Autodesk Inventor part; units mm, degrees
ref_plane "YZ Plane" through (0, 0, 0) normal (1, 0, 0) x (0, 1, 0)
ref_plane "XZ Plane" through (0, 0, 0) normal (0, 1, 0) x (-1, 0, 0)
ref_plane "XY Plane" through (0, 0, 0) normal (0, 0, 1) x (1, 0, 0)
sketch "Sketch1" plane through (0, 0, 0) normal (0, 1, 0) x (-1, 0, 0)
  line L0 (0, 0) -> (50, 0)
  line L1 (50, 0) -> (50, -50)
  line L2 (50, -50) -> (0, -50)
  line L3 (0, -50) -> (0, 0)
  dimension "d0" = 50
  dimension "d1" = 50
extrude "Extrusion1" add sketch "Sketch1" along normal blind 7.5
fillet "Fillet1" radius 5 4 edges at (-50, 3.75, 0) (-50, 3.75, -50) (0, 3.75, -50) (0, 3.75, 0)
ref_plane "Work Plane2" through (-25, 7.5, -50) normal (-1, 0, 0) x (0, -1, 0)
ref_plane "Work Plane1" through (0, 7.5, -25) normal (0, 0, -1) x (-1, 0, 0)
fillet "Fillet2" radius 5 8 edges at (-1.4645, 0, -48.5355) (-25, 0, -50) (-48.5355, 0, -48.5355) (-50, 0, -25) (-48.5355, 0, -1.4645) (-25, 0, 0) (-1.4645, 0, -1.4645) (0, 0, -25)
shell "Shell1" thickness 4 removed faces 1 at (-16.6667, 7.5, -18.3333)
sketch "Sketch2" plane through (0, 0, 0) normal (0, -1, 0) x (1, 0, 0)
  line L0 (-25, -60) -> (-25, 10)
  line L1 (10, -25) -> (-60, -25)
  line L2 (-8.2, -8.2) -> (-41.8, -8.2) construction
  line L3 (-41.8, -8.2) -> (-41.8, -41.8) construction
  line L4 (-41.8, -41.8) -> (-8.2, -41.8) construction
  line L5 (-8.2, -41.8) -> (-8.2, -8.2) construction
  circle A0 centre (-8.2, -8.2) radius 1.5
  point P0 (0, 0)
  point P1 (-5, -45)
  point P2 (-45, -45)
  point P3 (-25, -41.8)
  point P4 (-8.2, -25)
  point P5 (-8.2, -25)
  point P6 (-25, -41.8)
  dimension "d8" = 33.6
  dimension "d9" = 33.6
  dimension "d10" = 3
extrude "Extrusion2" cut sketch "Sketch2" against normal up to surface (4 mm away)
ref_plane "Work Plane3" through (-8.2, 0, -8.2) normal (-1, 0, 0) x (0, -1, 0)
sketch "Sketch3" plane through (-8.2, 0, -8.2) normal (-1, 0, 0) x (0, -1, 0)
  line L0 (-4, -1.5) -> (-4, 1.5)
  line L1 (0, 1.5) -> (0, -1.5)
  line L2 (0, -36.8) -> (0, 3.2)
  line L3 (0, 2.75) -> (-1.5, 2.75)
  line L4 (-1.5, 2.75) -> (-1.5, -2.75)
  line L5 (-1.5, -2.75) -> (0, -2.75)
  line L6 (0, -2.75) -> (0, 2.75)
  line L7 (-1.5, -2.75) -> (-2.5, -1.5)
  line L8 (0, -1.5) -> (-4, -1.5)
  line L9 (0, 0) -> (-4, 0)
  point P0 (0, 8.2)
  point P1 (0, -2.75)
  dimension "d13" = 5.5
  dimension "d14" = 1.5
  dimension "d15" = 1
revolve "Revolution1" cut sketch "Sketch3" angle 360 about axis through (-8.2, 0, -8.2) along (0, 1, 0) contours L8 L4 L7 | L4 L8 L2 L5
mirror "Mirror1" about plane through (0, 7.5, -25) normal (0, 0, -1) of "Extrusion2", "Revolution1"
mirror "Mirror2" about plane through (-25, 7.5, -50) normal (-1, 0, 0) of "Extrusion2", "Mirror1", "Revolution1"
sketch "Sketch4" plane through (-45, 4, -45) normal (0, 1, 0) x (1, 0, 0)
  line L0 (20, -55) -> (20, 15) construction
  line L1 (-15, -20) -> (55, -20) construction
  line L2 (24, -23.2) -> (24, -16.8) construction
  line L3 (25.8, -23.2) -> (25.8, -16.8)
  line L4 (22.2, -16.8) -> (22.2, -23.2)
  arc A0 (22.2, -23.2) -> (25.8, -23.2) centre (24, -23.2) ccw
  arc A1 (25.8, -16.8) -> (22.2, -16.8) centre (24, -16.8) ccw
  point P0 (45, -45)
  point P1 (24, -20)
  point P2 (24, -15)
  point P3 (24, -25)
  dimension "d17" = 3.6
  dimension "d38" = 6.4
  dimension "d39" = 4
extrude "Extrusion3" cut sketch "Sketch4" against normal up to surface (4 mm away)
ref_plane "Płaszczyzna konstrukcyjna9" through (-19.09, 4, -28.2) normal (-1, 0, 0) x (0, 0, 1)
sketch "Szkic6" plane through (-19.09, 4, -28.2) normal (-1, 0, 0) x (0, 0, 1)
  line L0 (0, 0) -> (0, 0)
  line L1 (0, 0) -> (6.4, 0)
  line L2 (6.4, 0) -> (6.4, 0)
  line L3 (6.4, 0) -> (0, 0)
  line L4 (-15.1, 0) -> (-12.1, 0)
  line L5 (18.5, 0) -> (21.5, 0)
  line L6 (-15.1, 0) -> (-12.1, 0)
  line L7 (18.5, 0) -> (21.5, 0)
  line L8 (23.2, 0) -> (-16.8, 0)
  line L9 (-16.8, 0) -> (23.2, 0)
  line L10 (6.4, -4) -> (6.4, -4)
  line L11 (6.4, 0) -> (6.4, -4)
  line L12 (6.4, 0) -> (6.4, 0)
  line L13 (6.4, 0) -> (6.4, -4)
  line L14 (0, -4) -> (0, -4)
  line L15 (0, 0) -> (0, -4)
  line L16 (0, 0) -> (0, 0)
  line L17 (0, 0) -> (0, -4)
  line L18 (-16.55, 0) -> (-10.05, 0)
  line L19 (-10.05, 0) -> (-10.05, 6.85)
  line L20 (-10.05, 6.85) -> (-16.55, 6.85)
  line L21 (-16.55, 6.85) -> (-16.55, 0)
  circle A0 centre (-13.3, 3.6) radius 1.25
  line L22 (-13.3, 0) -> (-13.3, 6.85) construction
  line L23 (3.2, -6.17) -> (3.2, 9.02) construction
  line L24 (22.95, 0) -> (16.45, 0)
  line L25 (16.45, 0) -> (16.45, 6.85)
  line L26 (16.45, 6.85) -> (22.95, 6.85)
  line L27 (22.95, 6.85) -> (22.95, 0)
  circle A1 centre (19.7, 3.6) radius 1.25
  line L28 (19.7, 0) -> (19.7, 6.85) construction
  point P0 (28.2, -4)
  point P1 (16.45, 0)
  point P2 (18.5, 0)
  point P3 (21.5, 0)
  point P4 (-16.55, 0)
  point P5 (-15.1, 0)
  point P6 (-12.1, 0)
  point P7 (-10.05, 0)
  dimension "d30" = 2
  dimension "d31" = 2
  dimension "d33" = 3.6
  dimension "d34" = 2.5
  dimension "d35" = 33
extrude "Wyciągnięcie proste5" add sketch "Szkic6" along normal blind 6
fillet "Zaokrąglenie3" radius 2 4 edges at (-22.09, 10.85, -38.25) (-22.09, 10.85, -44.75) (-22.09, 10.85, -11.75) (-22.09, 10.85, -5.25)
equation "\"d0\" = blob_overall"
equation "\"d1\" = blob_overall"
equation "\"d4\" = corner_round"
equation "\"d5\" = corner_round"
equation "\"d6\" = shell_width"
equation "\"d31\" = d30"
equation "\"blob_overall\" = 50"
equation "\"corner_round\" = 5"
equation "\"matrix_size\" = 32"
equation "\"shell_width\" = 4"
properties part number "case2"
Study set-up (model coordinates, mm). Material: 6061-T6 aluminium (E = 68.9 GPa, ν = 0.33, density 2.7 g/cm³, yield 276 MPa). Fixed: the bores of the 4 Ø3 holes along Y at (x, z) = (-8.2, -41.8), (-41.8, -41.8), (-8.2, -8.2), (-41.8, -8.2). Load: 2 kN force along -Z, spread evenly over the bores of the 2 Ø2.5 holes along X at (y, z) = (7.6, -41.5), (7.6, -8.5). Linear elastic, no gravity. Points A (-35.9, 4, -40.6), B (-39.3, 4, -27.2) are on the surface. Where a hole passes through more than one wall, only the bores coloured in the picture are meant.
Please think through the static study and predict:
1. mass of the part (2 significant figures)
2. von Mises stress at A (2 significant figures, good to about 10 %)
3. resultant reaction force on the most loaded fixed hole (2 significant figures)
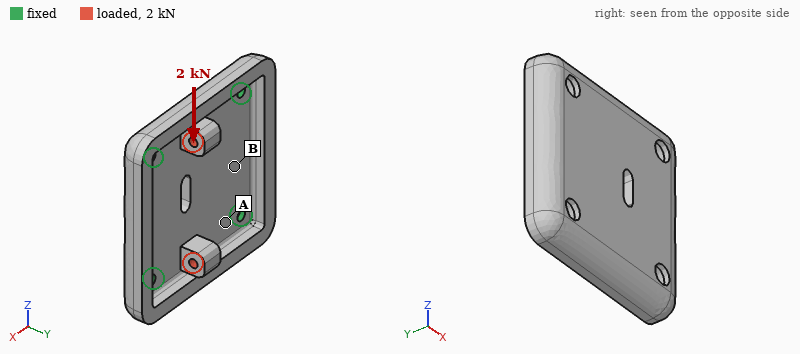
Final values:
31 g
28 MPa
590 N
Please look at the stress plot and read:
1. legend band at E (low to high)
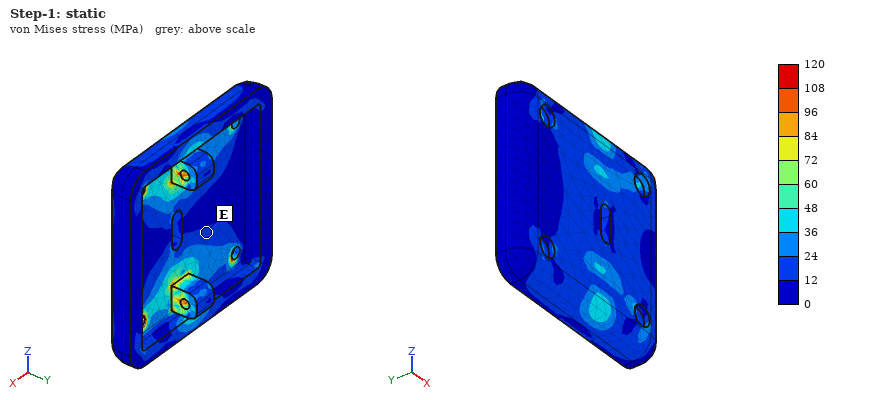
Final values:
12 to 24 MPa
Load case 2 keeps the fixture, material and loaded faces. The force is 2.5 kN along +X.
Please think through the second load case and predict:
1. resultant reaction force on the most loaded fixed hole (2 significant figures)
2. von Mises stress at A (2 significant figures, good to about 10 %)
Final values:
740 N
20 MPa
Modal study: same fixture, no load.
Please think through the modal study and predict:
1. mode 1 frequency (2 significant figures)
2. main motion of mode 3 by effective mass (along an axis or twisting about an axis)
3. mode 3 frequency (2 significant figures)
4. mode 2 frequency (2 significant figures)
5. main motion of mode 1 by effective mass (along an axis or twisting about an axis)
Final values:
10 kHz
twisting about X
13 kHz
11 kHz
along Y
